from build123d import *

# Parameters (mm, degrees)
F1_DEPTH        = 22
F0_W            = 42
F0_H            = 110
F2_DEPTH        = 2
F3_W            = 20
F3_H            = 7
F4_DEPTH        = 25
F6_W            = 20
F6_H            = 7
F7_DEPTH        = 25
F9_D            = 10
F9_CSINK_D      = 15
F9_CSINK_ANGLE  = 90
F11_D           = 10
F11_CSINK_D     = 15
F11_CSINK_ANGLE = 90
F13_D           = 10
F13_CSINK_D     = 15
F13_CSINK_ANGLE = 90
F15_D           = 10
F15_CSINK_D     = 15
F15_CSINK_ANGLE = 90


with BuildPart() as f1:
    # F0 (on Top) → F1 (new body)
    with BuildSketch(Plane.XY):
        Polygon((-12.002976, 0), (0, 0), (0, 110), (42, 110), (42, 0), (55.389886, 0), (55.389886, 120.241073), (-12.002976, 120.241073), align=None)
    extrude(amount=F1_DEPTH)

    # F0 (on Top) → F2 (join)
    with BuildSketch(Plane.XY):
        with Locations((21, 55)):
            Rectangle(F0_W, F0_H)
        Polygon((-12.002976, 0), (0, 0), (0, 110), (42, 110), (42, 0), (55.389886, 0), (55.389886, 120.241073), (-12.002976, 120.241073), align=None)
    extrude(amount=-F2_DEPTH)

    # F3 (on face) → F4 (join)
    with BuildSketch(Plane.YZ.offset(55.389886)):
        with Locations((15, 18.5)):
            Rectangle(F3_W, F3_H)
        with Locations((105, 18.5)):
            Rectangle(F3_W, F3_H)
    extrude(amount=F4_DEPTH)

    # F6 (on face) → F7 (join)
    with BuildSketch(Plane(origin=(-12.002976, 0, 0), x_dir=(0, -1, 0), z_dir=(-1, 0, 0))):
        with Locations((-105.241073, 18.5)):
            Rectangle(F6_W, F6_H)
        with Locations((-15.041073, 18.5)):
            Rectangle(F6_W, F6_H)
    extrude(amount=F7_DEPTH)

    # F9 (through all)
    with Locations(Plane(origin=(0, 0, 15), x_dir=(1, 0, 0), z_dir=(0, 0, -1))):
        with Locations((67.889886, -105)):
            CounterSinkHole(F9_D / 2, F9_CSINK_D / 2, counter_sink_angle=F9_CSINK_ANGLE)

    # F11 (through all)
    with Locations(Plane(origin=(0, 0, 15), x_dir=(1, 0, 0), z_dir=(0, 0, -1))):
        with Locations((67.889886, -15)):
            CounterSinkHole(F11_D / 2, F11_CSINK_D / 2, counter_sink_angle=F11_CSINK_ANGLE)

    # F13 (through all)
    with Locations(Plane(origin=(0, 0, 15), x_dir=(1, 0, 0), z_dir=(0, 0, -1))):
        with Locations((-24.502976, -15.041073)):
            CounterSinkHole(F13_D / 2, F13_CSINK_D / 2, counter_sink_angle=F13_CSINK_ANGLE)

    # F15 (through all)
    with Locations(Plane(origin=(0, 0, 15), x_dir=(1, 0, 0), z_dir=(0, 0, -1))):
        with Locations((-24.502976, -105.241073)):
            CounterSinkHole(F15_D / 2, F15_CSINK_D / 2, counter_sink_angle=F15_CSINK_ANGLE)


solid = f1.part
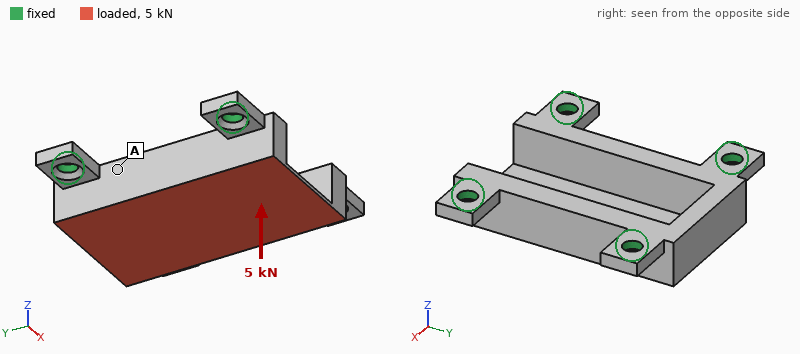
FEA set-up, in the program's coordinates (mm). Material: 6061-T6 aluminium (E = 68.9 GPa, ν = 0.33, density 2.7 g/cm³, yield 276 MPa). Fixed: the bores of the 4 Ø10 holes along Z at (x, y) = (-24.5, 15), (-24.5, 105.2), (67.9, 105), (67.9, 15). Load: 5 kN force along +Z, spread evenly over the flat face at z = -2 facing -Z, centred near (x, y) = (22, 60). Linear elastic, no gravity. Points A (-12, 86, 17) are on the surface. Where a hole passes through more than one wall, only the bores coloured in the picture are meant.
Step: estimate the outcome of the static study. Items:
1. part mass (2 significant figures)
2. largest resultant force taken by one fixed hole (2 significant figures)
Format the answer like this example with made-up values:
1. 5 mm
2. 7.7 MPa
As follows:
1. 280 g
2. 1.8 kN
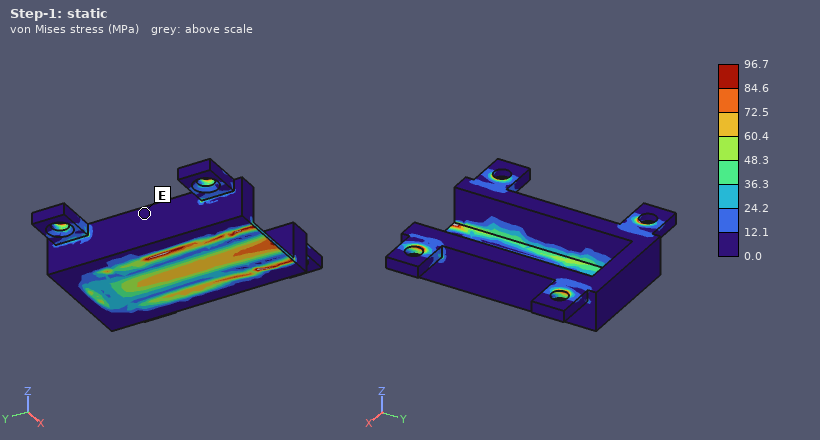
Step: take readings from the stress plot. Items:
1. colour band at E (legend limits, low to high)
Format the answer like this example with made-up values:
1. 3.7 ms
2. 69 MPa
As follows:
1. 0.0 to 12.1 MPa
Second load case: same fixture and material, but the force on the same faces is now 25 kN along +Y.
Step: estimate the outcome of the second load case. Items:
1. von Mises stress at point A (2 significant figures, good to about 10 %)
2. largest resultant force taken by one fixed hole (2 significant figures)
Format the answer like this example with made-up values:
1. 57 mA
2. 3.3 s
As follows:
1. 57 MPa
2. 7.3 kN
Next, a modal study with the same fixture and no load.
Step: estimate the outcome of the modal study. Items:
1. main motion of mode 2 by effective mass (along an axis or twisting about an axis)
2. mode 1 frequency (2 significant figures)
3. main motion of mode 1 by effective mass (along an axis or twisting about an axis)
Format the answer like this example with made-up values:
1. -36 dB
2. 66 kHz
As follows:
1. along Z
2. 3300 Hz
3. along X
